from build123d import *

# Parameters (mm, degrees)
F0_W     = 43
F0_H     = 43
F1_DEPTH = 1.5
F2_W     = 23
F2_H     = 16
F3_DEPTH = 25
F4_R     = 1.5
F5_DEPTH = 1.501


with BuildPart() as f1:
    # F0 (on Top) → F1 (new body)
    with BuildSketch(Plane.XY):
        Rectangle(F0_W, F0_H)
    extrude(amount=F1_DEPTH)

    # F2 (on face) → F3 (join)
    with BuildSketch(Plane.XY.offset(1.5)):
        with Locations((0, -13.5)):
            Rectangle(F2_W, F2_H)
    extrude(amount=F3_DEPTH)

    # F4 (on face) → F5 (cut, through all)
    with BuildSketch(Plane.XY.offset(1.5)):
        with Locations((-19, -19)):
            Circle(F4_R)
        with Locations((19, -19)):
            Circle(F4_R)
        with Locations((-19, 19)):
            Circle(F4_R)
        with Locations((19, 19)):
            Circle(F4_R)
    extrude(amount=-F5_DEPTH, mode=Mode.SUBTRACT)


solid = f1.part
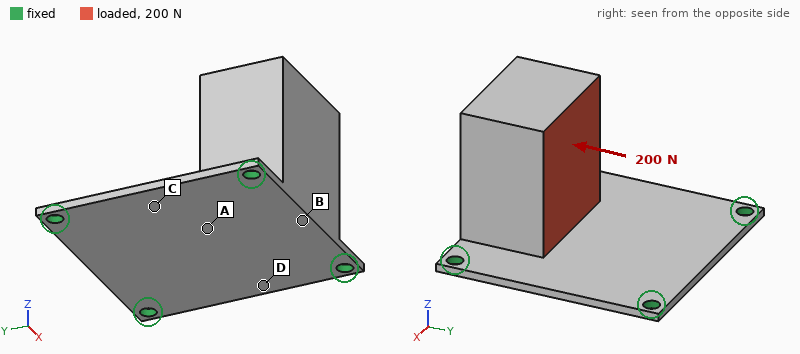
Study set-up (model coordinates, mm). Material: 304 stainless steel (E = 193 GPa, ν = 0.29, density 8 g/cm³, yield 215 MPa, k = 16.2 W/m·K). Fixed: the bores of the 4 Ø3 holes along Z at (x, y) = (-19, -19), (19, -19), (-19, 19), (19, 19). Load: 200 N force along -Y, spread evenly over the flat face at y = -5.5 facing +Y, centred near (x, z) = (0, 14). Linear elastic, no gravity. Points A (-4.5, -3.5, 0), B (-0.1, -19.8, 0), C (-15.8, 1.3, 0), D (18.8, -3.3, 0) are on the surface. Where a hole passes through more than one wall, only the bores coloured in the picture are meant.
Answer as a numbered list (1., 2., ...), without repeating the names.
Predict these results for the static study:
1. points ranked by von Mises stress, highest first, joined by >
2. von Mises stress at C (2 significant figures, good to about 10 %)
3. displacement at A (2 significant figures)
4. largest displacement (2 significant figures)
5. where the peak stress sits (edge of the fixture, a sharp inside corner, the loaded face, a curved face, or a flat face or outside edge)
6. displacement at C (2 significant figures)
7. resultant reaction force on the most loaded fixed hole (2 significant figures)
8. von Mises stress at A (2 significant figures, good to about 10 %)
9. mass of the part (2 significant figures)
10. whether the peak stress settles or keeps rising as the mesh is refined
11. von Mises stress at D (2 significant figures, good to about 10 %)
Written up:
1. A > D > C > B
2. 32 MPa
3. 29 µm
4. 68 µm
5. edge of the fixture
6. 24 µm
7. 80 N
8. 56 MPa
9. 95 g
10. keeps rising
11. 41 MPa
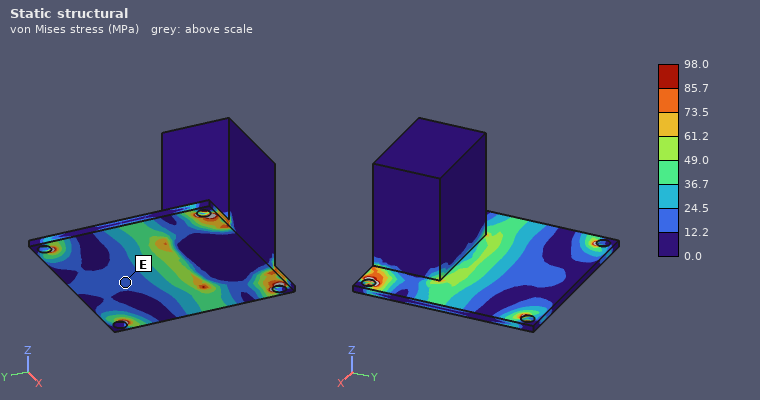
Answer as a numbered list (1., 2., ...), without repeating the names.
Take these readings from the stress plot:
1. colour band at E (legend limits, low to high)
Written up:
1. 12.2 to 24.5 MPa
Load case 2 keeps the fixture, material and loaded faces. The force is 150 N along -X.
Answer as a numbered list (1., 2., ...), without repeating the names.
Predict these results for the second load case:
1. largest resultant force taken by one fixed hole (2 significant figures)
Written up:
1. 89 N
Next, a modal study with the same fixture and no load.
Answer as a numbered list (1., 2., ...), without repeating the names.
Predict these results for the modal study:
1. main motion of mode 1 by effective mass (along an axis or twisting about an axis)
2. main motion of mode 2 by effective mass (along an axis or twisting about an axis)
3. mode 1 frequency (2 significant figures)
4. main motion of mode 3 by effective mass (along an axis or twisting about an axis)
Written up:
1. along Y
2. along X
3. 1200 Hz
4. along Z
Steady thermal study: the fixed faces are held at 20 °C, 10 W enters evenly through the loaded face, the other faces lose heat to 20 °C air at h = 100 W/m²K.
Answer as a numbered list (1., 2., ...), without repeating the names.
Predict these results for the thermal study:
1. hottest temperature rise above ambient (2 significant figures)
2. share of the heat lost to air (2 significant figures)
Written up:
1. 40 K
2. 86 %
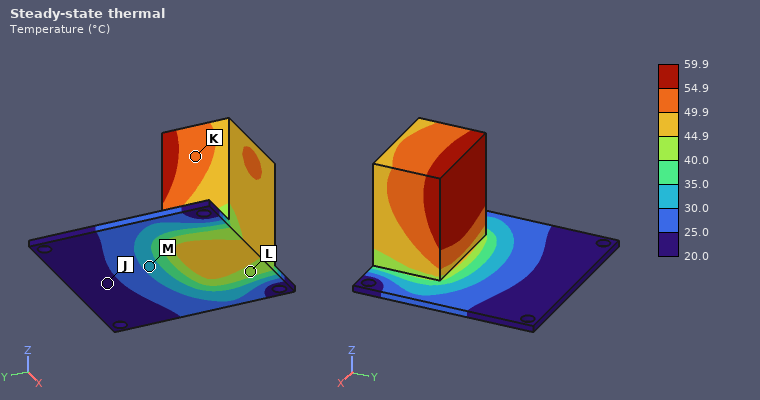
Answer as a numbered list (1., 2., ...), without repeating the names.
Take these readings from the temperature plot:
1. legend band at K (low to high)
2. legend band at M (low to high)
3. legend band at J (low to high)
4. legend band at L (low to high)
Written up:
1. 49.9 to 54.9 °C
2. 30.0 to 35.0 °C
3. 20.0 to 25.0 °C
4. 40.0 to 44.9 °C
